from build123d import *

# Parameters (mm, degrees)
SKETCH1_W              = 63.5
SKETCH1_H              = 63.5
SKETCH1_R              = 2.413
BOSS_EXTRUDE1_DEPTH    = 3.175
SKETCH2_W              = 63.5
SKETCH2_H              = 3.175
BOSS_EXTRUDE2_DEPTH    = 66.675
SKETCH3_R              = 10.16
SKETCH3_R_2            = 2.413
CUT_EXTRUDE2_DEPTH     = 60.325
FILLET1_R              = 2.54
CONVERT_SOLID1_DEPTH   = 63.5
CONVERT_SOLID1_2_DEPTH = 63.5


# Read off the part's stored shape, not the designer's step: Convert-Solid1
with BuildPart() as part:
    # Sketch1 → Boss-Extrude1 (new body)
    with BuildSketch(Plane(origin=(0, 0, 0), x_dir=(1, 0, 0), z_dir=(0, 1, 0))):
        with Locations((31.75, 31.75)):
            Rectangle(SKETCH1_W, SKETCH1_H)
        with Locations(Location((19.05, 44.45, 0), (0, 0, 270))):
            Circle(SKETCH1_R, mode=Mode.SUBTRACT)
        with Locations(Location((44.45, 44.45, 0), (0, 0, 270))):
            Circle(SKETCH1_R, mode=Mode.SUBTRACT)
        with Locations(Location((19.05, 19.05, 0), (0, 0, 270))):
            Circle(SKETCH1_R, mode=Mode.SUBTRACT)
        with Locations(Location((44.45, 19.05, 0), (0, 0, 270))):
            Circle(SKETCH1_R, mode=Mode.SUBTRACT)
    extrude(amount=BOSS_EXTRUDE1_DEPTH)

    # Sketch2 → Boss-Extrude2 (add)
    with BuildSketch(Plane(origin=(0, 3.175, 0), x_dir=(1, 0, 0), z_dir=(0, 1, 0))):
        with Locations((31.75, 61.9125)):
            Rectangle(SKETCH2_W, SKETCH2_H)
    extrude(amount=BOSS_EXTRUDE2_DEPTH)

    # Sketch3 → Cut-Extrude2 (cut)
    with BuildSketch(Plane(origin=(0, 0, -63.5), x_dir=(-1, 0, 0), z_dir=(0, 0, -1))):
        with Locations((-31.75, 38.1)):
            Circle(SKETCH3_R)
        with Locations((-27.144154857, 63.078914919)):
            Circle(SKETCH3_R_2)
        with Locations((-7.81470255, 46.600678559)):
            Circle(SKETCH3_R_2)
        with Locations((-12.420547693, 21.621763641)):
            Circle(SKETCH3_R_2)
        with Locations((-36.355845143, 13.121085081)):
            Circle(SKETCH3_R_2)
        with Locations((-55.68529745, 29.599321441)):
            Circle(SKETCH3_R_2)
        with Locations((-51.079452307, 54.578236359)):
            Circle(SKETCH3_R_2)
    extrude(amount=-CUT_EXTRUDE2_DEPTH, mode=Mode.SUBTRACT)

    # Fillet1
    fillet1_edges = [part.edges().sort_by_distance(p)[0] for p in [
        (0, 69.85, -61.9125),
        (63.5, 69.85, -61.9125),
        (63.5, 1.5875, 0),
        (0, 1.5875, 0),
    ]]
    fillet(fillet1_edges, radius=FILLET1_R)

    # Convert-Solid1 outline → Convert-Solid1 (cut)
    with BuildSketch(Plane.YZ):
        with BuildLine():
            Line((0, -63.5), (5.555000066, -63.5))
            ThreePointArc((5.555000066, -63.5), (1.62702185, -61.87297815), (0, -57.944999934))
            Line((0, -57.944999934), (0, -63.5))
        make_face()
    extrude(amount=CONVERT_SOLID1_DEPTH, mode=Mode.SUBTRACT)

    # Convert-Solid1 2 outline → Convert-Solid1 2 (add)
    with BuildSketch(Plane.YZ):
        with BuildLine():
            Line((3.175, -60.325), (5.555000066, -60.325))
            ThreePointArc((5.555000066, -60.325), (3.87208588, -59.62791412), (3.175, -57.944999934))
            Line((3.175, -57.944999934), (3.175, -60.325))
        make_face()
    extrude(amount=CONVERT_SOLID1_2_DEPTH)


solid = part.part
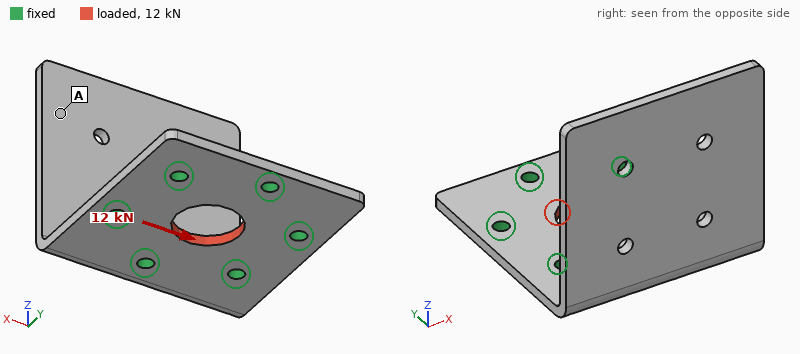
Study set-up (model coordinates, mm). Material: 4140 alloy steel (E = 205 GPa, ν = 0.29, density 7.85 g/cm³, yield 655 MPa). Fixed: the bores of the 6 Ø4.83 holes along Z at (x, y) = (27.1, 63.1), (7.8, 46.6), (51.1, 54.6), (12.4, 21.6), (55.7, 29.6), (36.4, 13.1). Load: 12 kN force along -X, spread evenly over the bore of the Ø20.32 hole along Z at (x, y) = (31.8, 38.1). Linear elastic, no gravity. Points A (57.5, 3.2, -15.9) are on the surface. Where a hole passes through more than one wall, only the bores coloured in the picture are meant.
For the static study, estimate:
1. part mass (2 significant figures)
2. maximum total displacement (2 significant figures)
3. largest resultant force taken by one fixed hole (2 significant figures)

190 g
5.1 µm
2.8 kN
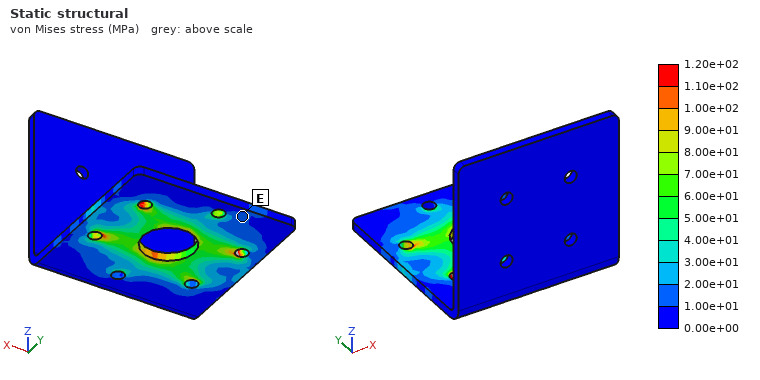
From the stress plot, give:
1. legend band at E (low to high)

1.00e+01 to 2.00e+01 MPa
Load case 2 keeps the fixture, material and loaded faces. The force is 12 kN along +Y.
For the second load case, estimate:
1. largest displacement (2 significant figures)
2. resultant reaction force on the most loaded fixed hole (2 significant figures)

5.0 µm
2.9 kN
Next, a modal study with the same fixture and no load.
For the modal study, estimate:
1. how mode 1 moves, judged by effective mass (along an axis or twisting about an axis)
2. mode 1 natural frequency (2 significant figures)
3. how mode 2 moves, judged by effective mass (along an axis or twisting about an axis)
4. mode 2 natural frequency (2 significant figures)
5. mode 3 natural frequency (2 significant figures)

along Y
530 Hz
along X
1100 Hz
1700 Hz
